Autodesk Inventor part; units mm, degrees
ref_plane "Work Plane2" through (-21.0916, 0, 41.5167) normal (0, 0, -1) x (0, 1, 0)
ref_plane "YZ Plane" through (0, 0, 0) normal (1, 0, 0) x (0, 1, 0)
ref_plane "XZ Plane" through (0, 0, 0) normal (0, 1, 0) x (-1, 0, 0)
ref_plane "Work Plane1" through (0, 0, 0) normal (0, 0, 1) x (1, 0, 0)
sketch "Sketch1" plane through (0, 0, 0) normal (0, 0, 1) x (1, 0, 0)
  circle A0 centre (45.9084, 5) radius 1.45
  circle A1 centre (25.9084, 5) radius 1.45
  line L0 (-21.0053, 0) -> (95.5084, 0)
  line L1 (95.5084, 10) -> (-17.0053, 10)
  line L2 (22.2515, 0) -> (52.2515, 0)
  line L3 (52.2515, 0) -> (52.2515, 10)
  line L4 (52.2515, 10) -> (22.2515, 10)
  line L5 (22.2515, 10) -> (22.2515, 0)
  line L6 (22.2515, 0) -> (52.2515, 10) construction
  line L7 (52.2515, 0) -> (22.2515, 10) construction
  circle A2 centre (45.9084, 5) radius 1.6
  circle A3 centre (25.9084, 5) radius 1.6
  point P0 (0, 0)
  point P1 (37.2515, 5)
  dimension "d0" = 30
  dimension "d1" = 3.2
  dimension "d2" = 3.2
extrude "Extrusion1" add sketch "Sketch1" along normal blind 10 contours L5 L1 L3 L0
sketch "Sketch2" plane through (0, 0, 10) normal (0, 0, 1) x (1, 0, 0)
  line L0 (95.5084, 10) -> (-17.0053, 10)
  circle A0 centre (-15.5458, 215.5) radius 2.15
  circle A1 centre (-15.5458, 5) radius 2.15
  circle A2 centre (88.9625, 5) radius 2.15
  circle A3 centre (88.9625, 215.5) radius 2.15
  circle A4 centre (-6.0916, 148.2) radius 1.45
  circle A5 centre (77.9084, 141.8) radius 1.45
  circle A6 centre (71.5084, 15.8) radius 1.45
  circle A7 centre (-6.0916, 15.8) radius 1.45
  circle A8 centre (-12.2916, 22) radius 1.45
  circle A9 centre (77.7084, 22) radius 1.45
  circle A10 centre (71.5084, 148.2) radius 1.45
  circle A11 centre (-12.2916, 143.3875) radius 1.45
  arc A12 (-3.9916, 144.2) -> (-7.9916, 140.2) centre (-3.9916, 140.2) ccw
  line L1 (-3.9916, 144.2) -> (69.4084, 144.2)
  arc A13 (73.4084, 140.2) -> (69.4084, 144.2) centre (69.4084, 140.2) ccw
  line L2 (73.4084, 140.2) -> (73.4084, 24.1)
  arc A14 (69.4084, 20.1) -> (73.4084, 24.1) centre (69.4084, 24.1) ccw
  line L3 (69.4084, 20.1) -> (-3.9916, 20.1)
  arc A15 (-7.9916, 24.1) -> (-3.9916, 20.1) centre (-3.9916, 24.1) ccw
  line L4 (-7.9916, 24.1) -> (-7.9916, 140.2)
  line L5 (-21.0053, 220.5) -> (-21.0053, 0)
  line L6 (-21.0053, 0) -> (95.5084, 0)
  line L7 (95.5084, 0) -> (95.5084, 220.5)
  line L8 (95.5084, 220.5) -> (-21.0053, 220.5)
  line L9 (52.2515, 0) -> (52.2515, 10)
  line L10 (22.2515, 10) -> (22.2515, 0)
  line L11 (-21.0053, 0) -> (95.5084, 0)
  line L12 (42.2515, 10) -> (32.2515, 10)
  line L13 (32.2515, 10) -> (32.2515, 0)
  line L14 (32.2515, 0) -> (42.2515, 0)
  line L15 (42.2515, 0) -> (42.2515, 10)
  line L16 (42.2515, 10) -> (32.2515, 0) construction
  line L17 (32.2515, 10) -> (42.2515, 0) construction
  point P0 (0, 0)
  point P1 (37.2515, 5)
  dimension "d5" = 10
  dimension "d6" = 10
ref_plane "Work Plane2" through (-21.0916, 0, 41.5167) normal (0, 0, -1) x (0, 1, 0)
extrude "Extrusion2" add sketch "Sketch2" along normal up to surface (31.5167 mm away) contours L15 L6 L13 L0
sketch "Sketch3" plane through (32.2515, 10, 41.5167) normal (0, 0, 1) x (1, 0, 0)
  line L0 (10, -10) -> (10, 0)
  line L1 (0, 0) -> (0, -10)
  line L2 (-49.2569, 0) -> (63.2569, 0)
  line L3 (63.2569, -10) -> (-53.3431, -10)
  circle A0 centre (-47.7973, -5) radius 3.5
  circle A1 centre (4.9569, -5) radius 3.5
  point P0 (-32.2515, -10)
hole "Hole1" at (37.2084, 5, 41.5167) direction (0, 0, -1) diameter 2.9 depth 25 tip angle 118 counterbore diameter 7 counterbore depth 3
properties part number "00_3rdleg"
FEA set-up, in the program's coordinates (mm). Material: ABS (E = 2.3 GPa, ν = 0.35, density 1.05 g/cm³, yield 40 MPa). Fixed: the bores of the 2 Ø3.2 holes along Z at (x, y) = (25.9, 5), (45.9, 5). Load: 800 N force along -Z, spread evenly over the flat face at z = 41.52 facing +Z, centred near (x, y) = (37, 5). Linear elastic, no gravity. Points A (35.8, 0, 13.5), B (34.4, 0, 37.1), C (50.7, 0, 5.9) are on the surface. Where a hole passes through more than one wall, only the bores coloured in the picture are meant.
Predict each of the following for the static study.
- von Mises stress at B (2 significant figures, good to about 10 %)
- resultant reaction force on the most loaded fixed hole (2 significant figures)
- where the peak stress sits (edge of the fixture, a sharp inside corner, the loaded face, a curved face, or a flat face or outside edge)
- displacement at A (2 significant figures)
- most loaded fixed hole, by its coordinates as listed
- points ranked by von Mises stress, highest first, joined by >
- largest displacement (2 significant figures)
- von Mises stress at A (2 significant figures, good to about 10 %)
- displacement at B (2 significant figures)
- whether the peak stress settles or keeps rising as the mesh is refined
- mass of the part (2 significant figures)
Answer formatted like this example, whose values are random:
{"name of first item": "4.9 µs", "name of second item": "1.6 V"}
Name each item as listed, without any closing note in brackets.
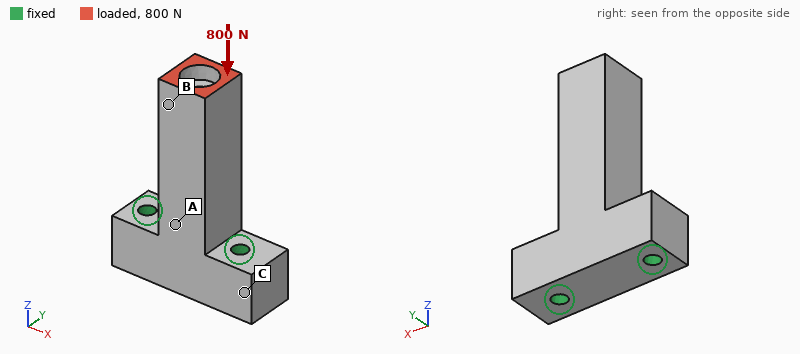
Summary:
{"von Mises stress at B": "12 MPa", "resultant reaction force on the most loaded fixed hole": "470 N", "where the peak stress sits": "edge of the fixture", "displacement at A": "0.058 mm", "most loaded fixed hole, by its coordinates as listed": "(45.9, 5)", "points ranked by von Mises stress, highest first, joined by >": "B > A > C", "largest displacement": "0.18 mm", "von Mises stress at A": "7.3 MPa", "displacement at B": "0.15 mm", "whether the peak stress settles or keeps rising as the mesh is refined": "keeps rising", "mass of the part": "6.0 g"}
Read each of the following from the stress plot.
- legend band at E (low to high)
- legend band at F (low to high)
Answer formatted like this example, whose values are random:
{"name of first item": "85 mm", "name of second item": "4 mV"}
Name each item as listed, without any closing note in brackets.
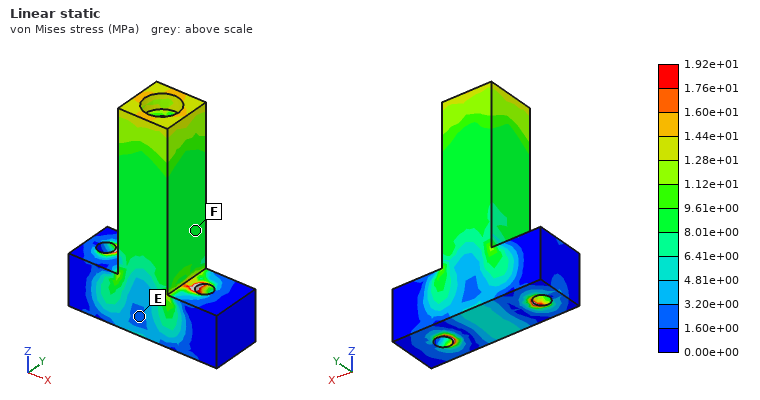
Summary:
{"legend band at E": "1.60e+00 to 3.20e+00 MPa", "legend band at F": "8.01e+00 to 9.61e+00 MPa"}
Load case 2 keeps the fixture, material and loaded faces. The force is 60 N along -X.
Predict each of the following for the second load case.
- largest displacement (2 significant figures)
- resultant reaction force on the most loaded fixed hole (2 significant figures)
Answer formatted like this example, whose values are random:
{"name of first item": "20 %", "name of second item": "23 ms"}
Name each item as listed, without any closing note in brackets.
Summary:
{"largest displacement": "0.49 mm", "resultant reaction force on the most loaded fixed hole": "130 N"}
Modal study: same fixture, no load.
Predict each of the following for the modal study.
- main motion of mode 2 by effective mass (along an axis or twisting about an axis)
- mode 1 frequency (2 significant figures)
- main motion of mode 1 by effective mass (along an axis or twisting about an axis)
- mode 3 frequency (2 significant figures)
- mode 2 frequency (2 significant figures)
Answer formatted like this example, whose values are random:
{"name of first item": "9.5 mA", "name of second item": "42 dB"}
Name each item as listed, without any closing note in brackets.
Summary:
{"main motion of mode 2 by effective mass": "along X", "mode 1 frequency": "1600 Hz", "main motion of mode 1 by effective mass": "along Y", "mode 3 frequency": "6200 Hz", "mode 2 frequency": "2000 Hz"}
